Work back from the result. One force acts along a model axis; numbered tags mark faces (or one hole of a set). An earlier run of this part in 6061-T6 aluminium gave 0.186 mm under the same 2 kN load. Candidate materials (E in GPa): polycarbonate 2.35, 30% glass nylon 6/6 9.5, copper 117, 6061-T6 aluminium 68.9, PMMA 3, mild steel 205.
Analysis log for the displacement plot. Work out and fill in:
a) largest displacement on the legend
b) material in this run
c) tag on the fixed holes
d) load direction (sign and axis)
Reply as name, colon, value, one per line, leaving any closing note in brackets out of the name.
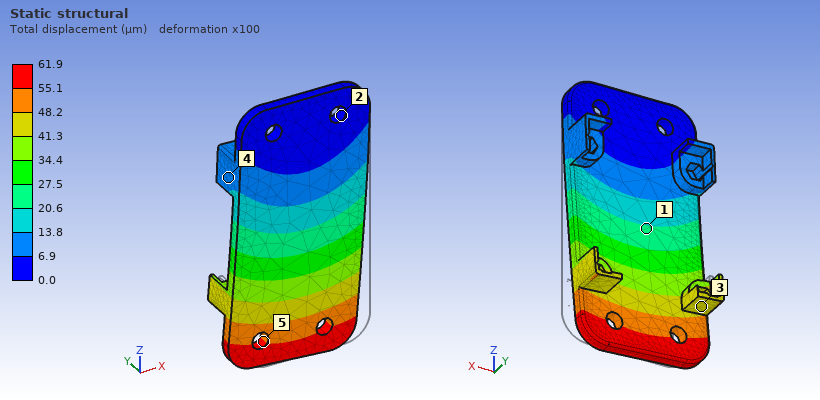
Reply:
largest displacement on the legend: 61.9 µm
material in this run: mild steel
tag on the fixed holes: 2
load direction: -X
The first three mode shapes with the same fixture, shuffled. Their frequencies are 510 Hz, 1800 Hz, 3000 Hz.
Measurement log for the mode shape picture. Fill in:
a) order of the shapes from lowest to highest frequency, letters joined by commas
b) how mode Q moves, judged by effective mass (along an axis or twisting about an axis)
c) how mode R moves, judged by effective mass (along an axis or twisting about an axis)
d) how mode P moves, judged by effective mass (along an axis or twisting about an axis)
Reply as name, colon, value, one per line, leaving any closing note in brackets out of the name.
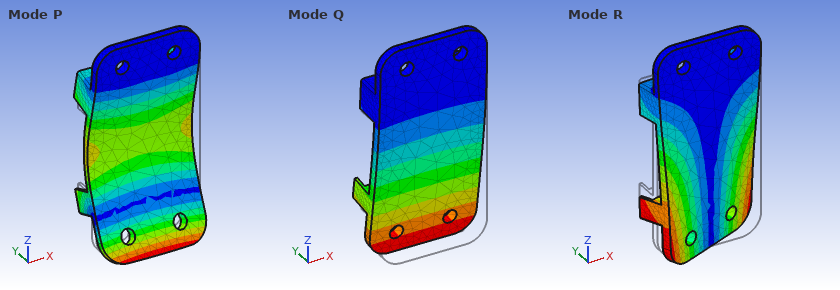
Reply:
order of the shapes from lowest to highest frequency, letters joined by commas: Q, R, P
how mode Q moves, judged by effective mass: along Y
how mode R moves, judged by effective mass: twisting about Z
how mode P moves, judged by effective mass: along Y
